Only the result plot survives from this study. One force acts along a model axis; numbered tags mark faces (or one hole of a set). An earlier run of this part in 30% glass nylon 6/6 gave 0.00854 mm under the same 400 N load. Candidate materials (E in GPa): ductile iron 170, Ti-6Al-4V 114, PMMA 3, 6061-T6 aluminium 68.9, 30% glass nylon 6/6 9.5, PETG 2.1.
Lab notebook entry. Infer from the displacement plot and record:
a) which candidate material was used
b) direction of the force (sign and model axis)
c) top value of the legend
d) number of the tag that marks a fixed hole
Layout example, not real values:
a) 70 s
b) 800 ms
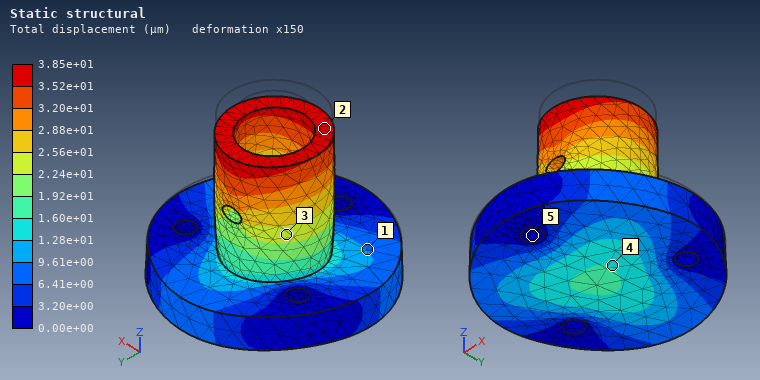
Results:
a) PETG
b) -Z
c) 3.85e+01 µm
d) 5
